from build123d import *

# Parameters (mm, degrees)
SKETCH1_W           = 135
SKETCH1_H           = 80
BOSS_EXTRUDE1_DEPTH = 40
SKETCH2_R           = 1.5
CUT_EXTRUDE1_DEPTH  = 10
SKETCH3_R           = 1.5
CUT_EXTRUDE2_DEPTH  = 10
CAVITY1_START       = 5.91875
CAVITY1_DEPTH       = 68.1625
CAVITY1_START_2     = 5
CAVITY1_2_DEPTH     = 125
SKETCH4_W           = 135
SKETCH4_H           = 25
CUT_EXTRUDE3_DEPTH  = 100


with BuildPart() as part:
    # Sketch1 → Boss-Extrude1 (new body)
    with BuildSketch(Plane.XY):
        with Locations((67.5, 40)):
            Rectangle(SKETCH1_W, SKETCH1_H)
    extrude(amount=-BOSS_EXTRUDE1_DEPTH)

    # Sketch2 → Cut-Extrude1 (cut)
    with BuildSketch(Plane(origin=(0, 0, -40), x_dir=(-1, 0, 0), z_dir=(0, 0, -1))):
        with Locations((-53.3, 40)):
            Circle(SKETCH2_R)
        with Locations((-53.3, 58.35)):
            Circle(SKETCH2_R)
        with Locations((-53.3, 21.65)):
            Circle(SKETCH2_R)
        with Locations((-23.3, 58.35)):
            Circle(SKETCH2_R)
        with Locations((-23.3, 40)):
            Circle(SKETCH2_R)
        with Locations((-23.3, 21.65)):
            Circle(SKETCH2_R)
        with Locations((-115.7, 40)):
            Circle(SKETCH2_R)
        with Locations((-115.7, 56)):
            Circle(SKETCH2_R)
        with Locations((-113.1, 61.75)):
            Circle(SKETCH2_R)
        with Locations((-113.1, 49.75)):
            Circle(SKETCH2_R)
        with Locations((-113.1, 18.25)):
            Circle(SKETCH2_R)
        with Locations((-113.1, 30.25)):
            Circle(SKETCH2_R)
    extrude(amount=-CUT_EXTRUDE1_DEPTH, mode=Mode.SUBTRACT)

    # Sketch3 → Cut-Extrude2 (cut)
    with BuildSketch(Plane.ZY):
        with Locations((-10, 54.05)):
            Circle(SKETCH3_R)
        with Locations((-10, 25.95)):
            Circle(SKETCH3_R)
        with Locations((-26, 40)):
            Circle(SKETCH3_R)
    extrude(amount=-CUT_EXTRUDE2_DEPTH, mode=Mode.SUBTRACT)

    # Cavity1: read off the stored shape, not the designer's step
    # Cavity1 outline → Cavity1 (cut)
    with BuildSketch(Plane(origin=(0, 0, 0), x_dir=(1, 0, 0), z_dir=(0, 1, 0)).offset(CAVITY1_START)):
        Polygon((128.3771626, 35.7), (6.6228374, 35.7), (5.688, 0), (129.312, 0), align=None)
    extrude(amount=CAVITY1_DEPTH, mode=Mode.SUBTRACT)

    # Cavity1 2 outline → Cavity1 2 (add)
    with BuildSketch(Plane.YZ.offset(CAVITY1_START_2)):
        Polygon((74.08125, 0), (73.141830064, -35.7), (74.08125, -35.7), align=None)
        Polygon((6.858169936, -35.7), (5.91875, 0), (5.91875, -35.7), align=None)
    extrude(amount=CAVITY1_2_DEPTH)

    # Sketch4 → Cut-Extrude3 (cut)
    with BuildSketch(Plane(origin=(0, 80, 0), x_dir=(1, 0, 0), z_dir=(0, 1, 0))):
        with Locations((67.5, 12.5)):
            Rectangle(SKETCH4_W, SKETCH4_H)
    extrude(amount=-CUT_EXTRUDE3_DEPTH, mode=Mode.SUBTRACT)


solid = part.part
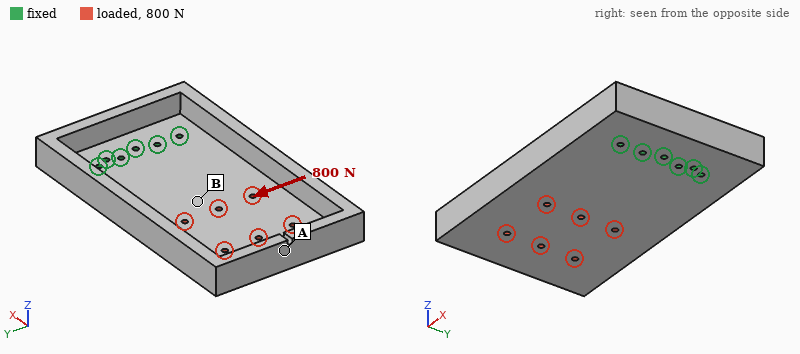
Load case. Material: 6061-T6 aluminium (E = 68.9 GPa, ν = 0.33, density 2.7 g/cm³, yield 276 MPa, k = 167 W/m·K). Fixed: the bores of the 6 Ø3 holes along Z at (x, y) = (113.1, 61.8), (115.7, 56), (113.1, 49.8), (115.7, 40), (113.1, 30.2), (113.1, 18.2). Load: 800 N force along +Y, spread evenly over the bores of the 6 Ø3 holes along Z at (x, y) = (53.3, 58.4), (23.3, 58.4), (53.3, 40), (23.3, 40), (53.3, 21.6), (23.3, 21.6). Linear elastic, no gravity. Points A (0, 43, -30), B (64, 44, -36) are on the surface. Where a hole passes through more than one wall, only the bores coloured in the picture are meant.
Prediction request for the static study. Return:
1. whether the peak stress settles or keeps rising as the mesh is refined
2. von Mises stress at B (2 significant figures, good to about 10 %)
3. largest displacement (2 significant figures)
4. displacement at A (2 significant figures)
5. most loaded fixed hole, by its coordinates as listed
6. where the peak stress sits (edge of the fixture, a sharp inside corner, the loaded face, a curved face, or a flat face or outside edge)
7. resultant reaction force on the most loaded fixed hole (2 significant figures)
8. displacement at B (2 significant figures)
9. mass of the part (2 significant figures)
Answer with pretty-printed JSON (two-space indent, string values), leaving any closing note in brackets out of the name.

{
  "whether the peak stress settles or keeps rising as the mesh is refined": "keeps rising",
  "von Mises stress at B": "6.6 MPa",
  "largest displacement": "40 µm",
  "displacement at A": "36 µm",
  "most loaded fixed hole, by its coordinates as listed": "(113.1, 18.2)",
  "where the peak stress sits": "edge of the fixture",
  "resultant reaction force on the most loaded fixed hole": "1.2 kN",
  "displacement at B": "15 µm",
  "mass of the part": "200 g"
}
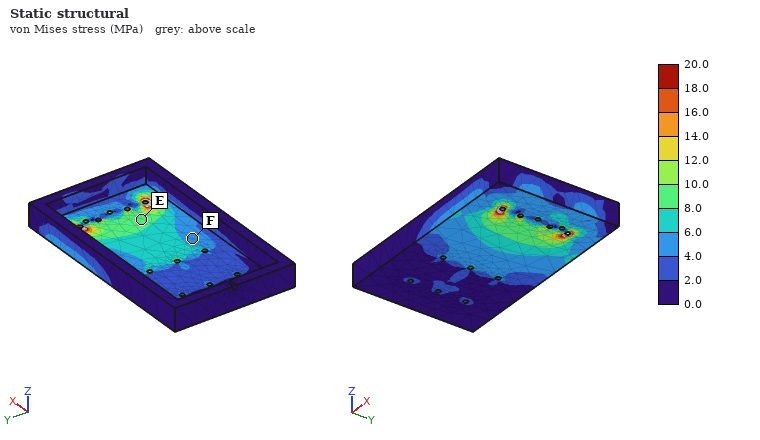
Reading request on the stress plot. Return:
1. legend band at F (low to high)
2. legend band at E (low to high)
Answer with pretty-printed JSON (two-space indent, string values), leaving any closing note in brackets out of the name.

{
  "legend band at F": "4.0 to 6.0 MPa",
  "legend band at E": "8.0 to 10.0 MPa"
}
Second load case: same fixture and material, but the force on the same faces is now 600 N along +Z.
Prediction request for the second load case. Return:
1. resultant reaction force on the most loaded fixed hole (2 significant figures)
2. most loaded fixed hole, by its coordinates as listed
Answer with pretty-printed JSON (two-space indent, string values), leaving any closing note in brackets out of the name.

{
  "resultant reaction force on the most loaded fixed hole": "1.0 kN",
  "most loaded fixed hole, by its coordinates as listed": "(113.1, 61.8)"
}
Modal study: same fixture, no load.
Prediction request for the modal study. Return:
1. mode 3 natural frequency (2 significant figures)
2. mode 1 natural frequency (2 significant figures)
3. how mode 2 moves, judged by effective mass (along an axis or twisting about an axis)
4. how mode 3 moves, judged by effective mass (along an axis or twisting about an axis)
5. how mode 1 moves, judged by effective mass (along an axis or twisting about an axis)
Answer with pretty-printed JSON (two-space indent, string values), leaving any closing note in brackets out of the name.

{
  "mode 3 natural frequency": "2400 Hz",
  "mode 1 natural frequency": "400 Hz",
  "how mode 2 moves, judged by effective mass": "twisting about X",
  "how mode 3 moves, judged by effective mass": "along Y",
  "how mode 1 moves, judged by effective mass": "along Z"
}
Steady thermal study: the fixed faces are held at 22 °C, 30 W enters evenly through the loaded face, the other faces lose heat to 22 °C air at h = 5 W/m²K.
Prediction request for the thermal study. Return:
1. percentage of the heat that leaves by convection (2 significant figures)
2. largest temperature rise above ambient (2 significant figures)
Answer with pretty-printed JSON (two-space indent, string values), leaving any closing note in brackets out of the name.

{
  "percentage of the heat that leaves by convection": "8.7 %",
  "largest temperature rise above ambient": "31 K"
}
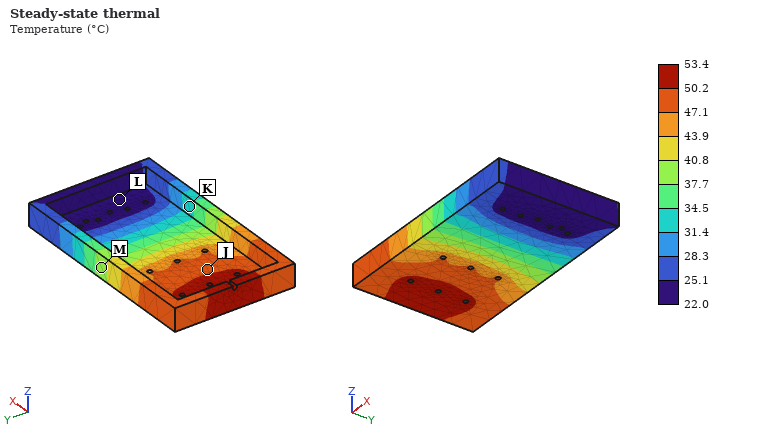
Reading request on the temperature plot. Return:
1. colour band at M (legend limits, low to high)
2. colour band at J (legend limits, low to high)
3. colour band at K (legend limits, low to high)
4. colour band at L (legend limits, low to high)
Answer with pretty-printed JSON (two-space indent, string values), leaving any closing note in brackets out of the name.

{
  "colour band at M": "37.7 to 40.8 °C",
  "colour band at J": "47.1 to 50.2 °C",
  "colour band at K": "31.4 to 34.5 °C",
  "colour band at L": "22.0 to 25.1 °C"
}
